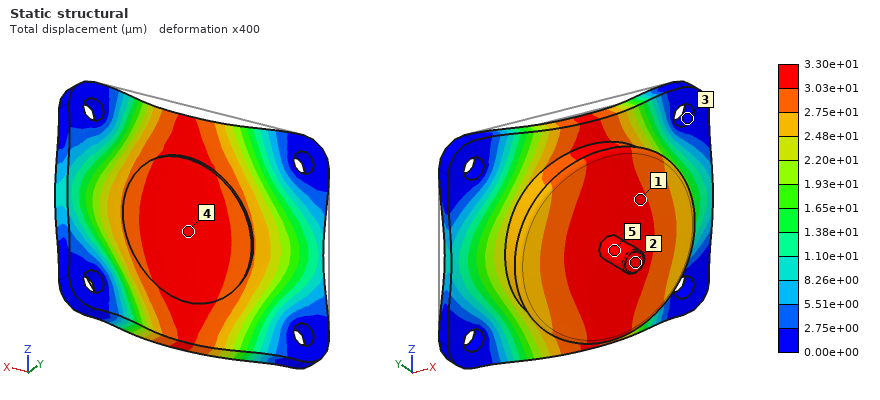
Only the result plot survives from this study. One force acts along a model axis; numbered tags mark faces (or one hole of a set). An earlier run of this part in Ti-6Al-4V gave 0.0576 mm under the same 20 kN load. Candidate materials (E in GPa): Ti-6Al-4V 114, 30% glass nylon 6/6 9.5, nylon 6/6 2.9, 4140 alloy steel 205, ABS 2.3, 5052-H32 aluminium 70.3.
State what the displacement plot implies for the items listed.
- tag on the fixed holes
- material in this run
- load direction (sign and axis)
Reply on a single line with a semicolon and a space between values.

3; 4140 alloy steel; -Y
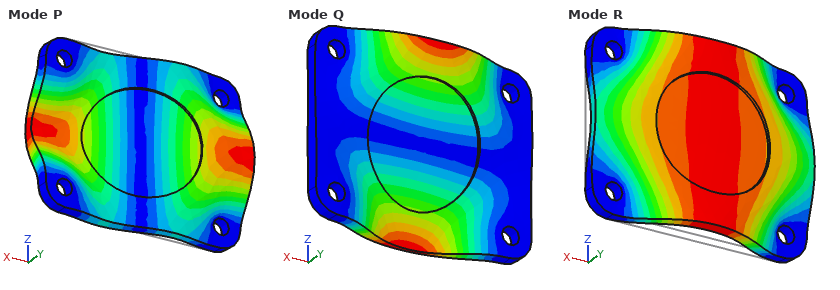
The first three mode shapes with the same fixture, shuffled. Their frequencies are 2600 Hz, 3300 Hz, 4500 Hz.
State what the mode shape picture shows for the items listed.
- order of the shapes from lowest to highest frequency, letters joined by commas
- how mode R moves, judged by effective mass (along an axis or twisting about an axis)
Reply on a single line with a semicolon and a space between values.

R, Q, P; along Y
